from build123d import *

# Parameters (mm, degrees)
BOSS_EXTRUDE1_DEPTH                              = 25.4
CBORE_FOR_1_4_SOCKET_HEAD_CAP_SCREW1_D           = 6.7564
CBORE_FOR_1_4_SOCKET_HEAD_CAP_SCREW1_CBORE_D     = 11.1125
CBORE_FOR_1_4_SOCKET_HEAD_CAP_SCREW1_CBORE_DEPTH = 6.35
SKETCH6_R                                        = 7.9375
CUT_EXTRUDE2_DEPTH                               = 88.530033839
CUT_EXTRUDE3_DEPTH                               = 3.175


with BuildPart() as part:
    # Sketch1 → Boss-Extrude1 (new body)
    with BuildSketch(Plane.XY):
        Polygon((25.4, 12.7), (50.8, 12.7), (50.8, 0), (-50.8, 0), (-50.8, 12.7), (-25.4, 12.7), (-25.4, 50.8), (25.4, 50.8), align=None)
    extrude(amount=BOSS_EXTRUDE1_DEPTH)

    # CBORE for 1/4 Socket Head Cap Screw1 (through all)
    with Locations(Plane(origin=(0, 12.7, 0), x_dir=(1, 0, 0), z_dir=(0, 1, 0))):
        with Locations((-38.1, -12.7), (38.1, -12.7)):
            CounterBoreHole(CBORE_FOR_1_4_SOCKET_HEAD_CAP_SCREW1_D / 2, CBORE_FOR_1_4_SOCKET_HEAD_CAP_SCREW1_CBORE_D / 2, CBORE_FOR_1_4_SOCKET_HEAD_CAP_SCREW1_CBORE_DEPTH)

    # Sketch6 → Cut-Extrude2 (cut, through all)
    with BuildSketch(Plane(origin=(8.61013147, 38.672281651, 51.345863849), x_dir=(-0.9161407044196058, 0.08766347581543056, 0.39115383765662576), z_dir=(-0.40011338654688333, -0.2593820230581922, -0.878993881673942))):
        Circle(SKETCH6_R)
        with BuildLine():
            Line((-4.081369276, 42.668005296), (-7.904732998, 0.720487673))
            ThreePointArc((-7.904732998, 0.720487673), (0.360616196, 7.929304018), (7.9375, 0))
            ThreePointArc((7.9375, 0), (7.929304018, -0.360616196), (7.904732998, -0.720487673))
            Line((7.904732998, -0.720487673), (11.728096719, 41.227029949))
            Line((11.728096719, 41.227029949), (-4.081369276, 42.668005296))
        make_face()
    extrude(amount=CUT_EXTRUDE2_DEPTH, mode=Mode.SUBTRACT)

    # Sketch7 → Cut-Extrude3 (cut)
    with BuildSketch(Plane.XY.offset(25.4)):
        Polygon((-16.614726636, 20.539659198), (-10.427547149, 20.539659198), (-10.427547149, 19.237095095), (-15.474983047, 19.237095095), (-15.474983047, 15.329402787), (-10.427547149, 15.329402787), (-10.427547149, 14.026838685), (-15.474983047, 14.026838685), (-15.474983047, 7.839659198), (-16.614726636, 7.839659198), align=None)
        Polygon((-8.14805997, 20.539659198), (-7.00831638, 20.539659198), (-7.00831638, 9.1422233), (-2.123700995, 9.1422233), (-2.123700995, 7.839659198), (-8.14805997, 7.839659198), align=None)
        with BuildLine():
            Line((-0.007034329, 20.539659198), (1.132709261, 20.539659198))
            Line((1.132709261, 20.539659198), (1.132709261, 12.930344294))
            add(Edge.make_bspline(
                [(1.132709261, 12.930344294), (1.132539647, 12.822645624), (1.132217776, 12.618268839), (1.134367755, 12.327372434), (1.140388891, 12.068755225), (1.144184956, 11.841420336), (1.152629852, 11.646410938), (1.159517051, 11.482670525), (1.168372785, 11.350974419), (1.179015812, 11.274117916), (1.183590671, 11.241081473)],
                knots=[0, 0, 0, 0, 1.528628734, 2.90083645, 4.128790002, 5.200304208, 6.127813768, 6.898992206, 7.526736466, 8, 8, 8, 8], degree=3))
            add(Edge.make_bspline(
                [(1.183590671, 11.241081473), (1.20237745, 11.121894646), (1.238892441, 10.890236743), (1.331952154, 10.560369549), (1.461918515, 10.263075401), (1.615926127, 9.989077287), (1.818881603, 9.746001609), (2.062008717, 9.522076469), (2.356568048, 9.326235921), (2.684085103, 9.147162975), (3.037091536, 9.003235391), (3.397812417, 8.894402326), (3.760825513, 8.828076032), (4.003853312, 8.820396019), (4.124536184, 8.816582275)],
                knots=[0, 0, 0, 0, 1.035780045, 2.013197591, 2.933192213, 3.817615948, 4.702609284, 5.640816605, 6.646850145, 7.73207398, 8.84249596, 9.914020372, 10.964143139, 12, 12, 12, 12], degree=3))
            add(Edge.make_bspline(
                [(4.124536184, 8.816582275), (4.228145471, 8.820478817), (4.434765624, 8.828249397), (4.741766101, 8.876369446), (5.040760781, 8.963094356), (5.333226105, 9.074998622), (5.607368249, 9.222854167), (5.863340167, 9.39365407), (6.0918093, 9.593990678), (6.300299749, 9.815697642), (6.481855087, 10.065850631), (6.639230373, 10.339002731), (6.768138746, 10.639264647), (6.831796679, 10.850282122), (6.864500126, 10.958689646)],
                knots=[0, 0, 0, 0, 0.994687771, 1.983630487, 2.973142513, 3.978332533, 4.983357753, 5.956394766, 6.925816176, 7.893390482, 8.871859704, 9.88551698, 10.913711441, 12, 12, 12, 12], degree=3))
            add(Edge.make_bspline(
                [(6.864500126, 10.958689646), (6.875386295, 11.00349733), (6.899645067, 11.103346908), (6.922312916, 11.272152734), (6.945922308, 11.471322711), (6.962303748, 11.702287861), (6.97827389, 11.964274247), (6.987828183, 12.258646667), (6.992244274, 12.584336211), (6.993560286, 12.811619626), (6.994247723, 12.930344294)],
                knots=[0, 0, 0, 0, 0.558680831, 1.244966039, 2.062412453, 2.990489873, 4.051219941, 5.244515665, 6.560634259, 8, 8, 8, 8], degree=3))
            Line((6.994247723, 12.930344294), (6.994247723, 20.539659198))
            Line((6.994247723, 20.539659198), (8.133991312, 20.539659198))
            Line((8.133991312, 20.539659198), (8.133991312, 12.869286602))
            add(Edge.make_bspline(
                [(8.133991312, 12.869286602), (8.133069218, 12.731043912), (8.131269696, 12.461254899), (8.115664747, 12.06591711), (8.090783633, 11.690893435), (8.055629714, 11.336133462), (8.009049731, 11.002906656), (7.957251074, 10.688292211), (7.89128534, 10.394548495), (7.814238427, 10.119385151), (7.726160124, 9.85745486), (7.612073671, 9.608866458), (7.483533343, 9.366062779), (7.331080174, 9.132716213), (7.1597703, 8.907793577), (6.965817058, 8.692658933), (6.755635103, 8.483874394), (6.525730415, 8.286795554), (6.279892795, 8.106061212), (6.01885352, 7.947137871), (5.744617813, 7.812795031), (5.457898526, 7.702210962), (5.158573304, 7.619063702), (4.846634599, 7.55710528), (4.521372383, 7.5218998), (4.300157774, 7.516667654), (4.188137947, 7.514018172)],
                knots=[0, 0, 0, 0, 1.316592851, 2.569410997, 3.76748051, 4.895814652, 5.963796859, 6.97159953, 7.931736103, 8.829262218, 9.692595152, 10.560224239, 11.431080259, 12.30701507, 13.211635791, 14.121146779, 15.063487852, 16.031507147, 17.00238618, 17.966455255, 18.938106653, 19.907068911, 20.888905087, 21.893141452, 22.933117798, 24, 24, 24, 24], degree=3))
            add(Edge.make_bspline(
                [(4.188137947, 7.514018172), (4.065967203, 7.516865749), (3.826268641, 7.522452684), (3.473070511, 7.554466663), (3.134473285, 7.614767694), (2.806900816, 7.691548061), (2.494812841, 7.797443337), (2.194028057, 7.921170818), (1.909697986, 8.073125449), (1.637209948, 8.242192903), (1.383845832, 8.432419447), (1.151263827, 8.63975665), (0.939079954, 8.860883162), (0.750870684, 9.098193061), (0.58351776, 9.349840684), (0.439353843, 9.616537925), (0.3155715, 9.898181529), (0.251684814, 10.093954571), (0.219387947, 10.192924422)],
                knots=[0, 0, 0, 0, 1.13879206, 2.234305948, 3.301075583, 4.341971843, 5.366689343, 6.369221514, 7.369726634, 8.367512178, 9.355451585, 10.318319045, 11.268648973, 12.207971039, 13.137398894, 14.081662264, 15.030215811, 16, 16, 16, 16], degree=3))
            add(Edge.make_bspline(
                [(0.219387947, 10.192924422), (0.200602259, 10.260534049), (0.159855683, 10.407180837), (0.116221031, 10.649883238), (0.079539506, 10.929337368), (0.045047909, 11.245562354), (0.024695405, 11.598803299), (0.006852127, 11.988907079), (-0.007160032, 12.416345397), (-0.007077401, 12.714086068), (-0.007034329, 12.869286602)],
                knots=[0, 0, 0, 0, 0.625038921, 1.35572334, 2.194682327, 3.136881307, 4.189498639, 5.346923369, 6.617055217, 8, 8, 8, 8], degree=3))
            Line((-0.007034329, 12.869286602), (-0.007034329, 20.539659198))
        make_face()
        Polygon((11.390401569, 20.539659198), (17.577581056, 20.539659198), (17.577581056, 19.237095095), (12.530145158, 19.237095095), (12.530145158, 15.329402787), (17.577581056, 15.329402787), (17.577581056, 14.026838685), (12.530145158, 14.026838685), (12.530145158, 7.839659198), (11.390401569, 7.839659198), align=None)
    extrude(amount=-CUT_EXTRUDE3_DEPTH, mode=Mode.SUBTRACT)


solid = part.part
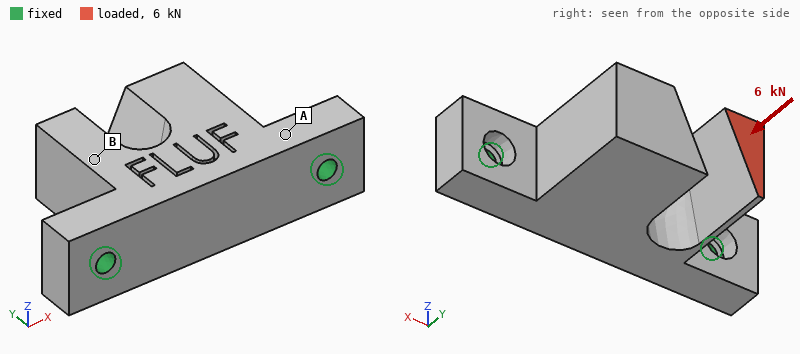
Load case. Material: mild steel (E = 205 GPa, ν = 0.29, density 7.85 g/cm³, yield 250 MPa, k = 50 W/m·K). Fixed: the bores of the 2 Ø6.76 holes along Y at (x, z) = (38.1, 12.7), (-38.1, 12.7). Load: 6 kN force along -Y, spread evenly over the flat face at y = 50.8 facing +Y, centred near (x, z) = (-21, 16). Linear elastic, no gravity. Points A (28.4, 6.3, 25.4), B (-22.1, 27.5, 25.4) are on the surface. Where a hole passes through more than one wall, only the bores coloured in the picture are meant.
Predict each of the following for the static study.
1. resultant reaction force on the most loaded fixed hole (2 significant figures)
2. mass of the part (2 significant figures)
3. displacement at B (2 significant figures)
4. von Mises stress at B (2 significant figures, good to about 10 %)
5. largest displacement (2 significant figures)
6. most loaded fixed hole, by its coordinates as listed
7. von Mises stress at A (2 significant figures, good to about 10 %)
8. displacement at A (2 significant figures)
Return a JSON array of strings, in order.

["5.3 kN", "520 g", "18 µm", "32 MPa", "27 µm", "(-38.1, 12.7)", "16 MPa", "4.5 µm"]
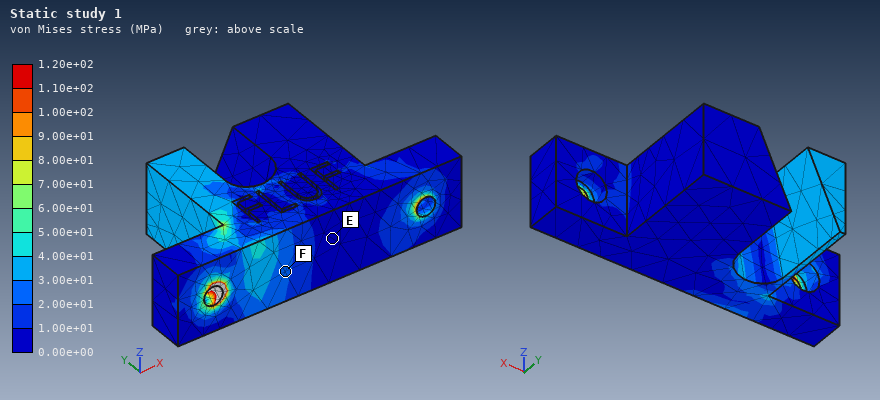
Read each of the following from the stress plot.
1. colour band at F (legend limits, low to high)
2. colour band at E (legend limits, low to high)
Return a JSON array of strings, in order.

["2.00e+01 to 3.00e+01 MPa", "0.00e+00 to 1.00e+01 MPa"]
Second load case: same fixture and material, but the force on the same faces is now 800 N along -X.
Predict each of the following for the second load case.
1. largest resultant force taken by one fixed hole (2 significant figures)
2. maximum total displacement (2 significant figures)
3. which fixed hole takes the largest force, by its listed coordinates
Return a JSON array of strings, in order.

["920 N", "42 µm", "(38.1, 12.7)"]
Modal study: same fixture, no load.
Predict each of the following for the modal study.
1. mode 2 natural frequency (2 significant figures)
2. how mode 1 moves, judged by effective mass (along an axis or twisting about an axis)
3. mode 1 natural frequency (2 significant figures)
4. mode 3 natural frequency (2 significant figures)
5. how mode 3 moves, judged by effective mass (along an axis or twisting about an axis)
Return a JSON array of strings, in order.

["5900 Hz", "along Z", "2400 Hz", "6700 Hz", "along Y"]
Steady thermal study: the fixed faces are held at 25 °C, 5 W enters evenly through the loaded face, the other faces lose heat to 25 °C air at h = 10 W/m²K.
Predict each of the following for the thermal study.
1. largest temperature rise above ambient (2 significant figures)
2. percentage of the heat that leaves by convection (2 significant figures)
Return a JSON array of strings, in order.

["21 K", "12 %"]
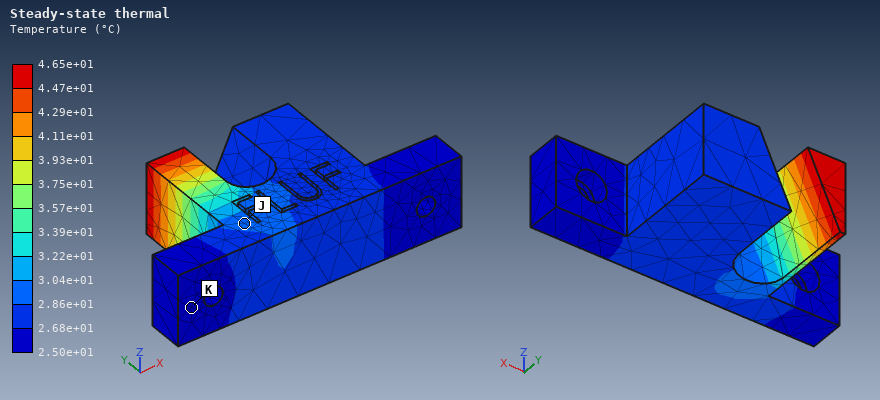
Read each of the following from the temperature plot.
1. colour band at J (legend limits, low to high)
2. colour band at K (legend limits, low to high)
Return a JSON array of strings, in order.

["2.86e+01 to 3.04e+01 °C", "2.50e+01 to 2.68e+01 °C"]
